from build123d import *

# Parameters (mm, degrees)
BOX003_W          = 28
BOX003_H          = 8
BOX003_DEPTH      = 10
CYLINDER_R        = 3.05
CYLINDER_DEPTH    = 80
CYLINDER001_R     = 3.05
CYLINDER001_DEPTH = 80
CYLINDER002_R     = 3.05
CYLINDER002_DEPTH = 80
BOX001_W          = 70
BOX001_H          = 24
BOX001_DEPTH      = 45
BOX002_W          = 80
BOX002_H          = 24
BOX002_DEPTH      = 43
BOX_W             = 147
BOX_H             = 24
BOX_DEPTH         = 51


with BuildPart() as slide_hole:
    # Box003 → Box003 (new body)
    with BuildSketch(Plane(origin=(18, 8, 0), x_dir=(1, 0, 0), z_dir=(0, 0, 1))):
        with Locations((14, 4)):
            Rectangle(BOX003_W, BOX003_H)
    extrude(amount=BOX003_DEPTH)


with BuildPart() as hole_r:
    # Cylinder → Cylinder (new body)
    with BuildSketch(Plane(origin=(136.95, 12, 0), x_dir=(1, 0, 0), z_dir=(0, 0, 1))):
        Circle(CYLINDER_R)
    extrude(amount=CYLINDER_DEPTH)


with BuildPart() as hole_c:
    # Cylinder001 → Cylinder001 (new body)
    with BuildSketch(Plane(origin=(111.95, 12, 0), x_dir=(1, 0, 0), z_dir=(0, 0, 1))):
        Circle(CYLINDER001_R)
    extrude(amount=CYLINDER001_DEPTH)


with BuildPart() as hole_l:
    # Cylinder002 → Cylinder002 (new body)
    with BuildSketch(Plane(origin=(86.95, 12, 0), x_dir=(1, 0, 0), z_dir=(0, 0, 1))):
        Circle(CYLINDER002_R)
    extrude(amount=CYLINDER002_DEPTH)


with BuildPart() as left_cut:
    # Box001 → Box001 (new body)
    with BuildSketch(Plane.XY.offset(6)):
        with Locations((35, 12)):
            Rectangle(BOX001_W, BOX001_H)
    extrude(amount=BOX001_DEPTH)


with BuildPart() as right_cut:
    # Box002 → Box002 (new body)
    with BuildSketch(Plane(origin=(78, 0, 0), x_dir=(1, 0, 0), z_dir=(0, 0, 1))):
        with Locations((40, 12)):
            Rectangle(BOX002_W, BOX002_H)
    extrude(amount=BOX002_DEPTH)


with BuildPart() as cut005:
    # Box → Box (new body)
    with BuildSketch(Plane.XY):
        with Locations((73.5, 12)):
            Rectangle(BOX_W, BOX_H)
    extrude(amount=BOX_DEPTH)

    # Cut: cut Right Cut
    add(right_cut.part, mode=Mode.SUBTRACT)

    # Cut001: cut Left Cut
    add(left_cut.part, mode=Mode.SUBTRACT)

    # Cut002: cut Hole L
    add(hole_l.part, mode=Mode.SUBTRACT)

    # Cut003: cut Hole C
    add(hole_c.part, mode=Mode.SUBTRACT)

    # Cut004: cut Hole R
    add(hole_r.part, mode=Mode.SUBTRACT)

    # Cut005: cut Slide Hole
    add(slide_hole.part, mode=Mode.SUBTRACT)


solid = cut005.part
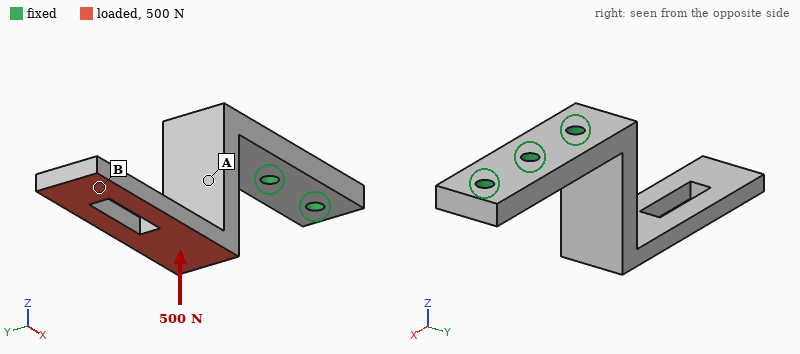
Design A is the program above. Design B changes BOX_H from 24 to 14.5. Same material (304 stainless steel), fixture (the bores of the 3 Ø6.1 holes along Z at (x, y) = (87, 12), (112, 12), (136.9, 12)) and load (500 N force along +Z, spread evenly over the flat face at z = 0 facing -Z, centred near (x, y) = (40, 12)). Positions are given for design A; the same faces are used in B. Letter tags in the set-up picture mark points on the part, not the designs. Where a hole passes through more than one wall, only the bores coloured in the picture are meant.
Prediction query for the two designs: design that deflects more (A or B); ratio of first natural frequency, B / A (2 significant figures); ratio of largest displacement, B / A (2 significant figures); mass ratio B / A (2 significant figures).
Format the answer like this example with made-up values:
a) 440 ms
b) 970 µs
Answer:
a) B
b) 1.0
c) 1.7
d) 0.58
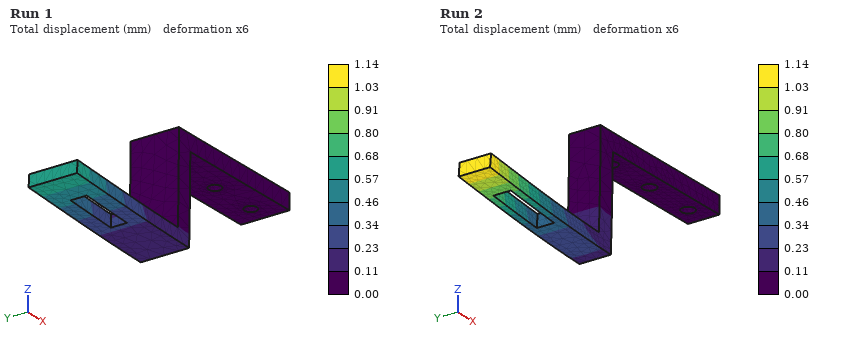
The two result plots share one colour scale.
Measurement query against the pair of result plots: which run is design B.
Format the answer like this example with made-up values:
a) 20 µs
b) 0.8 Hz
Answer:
a) Run 2
